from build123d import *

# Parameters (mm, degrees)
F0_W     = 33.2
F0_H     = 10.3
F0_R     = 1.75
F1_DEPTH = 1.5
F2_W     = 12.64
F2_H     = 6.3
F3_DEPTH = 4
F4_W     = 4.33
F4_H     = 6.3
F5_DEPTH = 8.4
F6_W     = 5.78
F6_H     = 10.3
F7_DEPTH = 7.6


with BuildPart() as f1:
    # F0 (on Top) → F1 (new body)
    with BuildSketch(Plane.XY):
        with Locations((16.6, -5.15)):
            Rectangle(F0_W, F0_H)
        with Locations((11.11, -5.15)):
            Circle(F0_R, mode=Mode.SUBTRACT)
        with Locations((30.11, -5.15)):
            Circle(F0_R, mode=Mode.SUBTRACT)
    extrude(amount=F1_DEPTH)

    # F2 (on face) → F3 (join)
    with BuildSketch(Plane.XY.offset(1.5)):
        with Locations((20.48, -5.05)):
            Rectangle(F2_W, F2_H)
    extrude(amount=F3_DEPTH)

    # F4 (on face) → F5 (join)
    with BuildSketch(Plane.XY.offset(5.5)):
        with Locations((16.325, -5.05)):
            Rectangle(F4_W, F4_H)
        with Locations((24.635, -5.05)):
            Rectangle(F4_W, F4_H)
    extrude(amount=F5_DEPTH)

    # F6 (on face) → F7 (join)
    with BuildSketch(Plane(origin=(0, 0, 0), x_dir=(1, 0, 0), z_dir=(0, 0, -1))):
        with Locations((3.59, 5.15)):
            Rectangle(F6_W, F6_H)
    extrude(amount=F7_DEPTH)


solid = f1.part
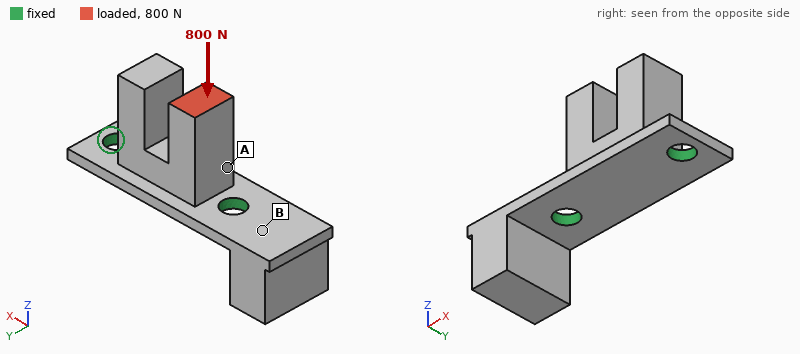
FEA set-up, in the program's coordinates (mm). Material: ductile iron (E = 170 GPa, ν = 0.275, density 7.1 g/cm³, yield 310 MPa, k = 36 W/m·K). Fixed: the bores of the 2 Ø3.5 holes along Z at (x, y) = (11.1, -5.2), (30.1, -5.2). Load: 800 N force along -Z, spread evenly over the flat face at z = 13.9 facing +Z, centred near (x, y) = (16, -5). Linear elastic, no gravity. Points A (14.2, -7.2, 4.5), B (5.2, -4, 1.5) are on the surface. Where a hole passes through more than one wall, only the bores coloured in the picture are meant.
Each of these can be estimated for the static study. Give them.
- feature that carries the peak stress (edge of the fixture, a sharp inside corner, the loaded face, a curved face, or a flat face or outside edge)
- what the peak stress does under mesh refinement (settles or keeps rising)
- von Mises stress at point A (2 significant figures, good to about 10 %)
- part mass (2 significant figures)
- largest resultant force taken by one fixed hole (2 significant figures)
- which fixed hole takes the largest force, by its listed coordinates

edge of the fixture
keeps rising
39 MPa
12 g
670 N
(11.1, -5.2)
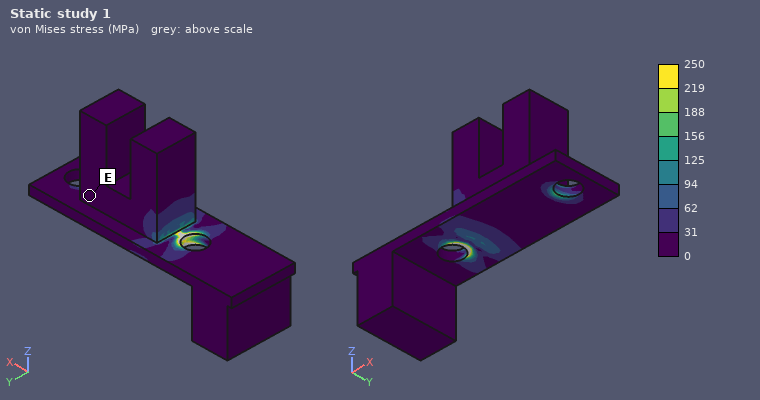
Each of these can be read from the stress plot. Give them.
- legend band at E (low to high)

0 to 31 MPa
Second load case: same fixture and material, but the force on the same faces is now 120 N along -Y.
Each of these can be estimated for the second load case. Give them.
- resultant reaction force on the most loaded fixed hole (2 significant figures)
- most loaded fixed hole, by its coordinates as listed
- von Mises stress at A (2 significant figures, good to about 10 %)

85 N
(11.1, -5.2)
27 MPa
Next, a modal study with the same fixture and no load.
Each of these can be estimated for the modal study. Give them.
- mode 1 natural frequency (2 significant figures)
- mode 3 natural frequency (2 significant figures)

4100 Hz
8000 Hz
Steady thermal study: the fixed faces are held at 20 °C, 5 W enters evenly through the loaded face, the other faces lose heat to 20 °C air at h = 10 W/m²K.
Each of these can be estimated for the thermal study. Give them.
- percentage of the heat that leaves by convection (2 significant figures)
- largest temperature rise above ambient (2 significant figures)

4.5 %
76 K
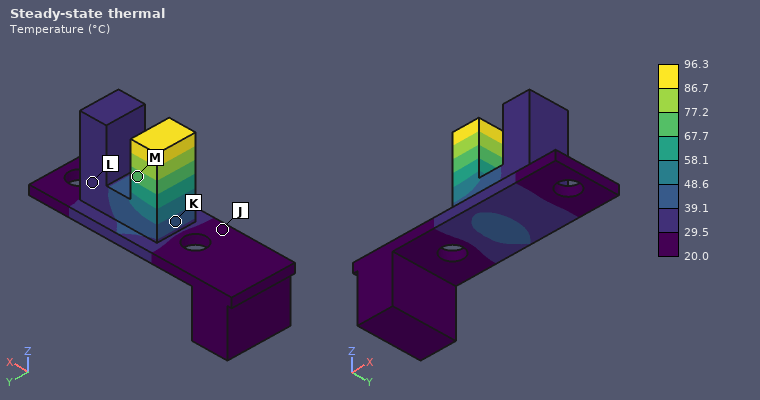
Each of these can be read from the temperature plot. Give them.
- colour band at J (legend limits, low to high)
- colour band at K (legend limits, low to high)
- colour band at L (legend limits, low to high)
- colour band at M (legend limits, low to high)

20.0 to 29.5 °C
39.1 to 48.6 °C
29.5 to 39.1 °C
67.7 to 77.2 °C
